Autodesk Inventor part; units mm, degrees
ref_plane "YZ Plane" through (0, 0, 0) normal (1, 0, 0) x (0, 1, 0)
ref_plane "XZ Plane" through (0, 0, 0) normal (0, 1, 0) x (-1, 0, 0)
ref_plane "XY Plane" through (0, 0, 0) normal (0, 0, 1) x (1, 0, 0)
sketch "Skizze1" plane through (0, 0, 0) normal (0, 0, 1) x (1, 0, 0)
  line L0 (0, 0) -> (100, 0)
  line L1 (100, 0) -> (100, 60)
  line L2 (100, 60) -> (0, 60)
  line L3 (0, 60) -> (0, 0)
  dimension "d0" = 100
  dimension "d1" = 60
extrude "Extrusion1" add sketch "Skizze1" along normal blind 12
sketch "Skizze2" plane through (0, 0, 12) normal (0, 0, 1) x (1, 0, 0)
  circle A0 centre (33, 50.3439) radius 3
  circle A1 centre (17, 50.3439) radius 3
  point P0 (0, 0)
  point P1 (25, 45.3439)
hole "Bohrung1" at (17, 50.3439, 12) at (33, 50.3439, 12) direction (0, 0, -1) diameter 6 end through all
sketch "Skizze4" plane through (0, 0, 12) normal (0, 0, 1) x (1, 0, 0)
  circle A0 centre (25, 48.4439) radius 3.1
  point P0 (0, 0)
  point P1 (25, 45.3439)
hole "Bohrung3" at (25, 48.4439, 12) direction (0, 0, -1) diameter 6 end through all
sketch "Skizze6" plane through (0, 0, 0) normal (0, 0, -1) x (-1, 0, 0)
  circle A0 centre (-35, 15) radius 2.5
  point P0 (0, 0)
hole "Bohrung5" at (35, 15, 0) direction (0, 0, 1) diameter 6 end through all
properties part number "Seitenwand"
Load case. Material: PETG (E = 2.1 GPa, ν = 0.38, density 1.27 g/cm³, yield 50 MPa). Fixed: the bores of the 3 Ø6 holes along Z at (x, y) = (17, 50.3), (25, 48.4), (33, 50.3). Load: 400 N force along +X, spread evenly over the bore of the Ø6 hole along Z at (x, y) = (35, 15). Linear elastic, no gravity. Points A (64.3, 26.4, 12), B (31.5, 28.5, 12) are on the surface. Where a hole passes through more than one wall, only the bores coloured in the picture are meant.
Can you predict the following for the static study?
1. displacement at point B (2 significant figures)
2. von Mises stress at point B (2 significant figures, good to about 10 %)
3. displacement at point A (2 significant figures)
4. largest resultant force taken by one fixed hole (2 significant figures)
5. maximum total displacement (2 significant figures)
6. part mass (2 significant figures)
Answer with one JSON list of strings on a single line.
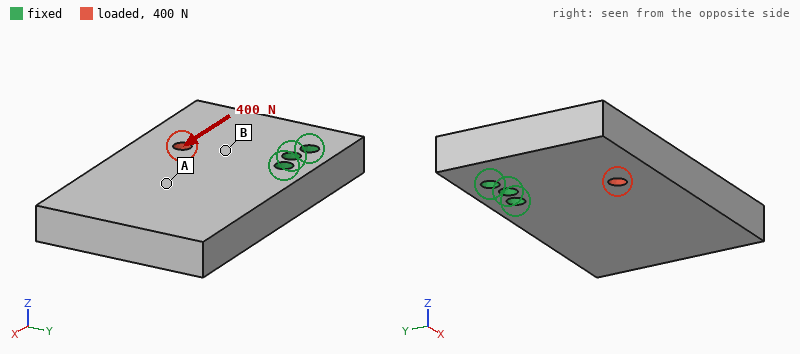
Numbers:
["0.064 mm", "1.8 MPa", "0.12 mm", "580 N", "0.25 mm", "90 g"]
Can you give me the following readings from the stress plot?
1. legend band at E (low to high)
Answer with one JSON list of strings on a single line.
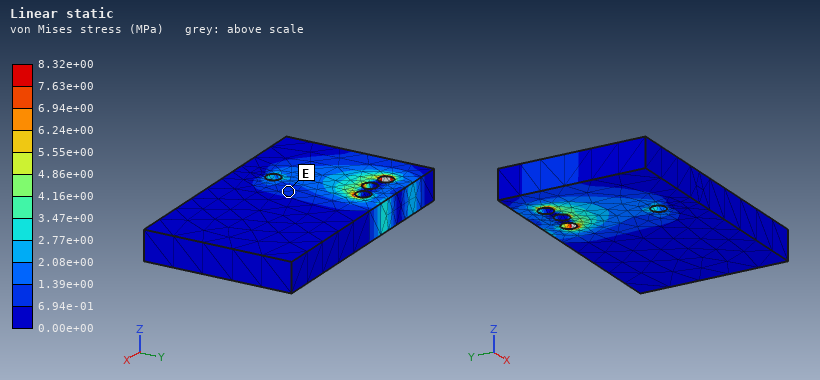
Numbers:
["6.94e-01 to 1.39e+00 MPa"]
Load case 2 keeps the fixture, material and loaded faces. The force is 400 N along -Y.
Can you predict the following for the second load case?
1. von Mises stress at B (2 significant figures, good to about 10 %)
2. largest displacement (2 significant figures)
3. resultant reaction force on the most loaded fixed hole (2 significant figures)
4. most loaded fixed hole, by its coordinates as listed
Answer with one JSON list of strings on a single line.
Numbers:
["1.4 MPa", "68 µm", "330 N", "(33, 50.3)"]
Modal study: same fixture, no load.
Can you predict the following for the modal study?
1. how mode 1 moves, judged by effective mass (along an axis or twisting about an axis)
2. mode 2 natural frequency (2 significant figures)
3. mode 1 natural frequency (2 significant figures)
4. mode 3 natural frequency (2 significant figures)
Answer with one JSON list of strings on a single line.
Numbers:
["along Z", "790 Hz", "410 Hz", "810 Hz"]
